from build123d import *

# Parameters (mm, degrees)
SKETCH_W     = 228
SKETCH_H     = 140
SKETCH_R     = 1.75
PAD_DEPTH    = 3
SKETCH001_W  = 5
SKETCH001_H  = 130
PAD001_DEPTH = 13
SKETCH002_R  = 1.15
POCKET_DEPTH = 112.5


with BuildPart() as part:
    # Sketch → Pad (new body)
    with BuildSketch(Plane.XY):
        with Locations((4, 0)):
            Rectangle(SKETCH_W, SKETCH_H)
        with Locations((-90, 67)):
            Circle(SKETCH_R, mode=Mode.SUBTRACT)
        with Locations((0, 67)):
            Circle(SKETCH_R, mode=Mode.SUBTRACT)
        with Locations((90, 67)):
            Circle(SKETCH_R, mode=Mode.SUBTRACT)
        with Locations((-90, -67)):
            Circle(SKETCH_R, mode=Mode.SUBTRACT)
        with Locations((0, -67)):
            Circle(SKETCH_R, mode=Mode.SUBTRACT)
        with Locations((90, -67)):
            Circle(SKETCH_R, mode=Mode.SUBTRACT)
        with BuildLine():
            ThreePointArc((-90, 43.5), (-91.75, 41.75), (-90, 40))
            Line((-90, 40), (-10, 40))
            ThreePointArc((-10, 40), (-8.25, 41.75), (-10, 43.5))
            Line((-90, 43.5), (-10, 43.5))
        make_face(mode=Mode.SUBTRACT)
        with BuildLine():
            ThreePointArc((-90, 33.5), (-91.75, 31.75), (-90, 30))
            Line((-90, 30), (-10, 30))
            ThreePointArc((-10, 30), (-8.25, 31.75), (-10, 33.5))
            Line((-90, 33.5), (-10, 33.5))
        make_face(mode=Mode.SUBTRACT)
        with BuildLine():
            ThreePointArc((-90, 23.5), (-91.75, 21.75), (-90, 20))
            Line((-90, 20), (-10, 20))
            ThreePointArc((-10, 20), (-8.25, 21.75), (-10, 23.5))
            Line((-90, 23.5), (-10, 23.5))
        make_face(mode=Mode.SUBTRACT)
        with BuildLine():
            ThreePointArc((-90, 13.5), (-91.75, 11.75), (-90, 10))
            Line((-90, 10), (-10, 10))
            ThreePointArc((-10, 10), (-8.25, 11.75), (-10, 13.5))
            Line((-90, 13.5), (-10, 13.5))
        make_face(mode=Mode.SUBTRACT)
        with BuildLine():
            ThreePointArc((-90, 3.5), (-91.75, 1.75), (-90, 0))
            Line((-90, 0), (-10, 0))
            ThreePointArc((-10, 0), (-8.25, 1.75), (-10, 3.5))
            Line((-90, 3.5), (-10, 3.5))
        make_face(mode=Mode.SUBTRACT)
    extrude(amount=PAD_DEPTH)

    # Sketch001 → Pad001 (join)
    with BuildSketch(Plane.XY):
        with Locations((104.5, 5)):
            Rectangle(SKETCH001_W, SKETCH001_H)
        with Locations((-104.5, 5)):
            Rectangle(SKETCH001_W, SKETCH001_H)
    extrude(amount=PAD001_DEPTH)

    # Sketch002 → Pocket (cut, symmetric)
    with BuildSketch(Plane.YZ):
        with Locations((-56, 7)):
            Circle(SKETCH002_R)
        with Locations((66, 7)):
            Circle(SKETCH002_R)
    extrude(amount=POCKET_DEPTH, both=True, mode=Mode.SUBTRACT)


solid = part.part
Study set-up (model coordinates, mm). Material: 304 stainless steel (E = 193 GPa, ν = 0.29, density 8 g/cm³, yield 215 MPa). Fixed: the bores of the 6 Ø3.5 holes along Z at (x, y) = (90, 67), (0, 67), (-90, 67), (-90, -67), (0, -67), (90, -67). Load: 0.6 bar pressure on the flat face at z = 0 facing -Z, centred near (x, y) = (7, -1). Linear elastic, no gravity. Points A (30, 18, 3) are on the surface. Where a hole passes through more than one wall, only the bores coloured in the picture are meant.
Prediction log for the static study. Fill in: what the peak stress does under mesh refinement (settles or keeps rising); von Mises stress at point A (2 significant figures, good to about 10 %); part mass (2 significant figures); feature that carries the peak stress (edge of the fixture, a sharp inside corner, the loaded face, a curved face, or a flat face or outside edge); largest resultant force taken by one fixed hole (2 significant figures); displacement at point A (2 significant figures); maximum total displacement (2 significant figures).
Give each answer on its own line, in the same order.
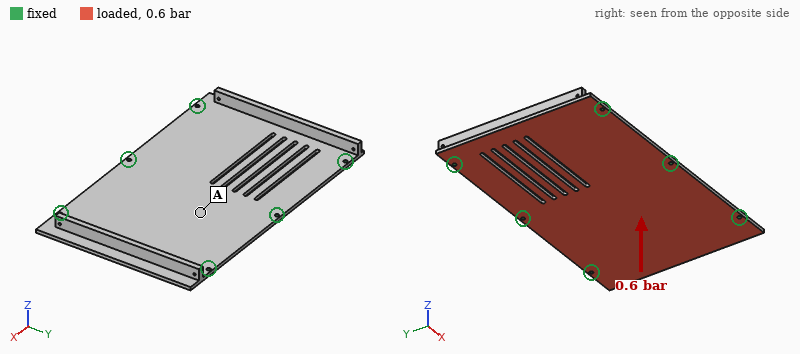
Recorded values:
keeps rising
30 MPa
830 g
edge of the fixture
420 N
0.17 mm
0.24 mm
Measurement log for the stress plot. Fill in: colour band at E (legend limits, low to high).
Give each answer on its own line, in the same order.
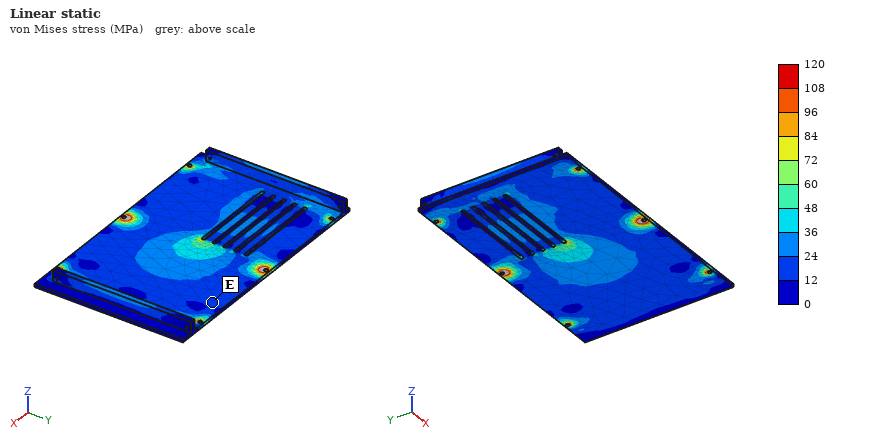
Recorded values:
12 to 24 MPa
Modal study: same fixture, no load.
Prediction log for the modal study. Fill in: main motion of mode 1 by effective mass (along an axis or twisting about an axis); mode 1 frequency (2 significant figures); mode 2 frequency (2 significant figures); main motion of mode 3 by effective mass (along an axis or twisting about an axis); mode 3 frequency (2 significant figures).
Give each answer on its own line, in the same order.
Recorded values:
along Z
660 Hz
950 Hz
along Z
1200 Hz
